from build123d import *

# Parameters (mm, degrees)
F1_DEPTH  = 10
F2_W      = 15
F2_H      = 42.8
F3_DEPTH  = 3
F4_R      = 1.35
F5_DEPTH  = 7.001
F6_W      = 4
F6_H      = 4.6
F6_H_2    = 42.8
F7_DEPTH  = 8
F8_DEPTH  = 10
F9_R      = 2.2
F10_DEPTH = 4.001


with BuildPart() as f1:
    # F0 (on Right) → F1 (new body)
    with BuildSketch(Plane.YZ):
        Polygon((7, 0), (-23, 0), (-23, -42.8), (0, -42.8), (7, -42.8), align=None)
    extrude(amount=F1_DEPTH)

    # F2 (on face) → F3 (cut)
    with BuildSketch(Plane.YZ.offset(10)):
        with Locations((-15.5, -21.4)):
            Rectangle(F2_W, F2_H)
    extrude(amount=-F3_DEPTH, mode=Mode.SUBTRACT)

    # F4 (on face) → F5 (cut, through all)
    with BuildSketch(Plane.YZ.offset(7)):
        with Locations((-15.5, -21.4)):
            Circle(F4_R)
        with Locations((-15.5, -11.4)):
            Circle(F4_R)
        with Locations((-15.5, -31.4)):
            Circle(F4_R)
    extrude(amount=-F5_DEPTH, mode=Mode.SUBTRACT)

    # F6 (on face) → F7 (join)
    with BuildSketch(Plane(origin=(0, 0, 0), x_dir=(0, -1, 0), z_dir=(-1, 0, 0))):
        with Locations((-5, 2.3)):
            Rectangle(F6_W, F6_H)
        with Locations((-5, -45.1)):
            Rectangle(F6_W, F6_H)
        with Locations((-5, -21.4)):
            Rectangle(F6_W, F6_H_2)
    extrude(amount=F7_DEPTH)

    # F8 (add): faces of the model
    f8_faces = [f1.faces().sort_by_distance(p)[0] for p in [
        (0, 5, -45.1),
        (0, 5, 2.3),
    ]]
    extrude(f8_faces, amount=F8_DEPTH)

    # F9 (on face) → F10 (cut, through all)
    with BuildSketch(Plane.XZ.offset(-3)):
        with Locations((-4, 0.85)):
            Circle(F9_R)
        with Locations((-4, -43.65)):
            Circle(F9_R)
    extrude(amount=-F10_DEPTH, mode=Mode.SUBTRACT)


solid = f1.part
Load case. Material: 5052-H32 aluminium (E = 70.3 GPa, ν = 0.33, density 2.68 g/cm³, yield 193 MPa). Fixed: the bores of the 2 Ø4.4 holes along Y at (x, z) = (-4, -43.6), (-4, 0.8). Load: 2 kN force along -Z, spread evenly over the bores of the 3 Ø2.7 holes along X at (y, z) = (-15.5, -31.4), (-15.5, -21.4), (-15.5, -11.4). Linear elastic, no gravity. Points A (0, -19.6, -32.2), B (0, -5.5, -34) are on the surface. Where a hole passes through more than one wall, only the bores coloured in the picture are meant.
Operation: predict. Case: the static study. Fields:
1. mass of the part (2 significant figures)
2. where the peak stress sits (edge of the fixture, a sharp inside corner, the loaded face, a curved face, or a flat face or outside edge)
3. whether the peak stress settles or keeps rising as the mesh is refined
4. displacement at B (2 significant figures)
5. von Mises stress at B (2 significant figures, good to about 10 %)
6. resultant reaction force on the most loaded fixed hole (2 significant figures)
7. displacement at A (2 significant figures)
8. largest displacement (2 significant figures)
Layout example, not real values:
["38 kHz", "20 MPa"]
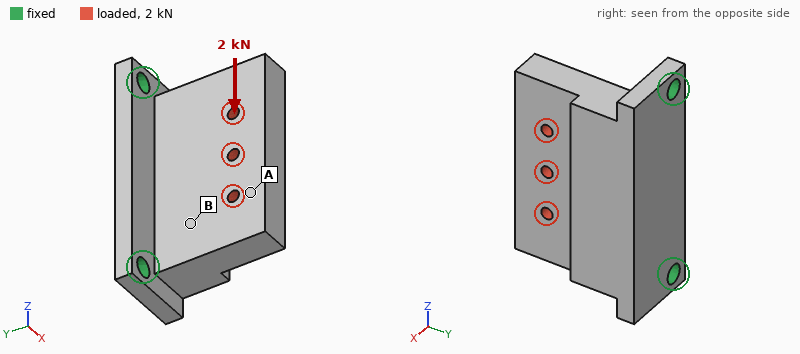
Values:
["34 g", "edge of the fixture", "keeps rising", "16 µm", "24 MPa", "1.4 kN", "29 µm", "36 µm"]
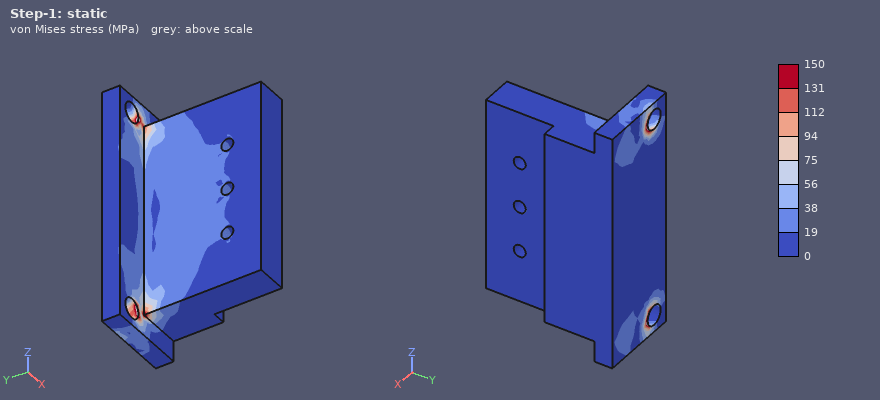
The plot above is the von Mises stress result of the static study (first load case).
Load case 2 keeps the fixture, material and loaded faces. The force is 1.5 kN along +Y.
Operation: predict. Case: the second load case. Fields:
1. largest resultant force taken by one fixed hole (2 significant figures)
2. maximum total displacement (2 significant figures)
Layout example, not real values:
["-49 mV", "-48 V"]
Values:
["770 N", "99 µm"]
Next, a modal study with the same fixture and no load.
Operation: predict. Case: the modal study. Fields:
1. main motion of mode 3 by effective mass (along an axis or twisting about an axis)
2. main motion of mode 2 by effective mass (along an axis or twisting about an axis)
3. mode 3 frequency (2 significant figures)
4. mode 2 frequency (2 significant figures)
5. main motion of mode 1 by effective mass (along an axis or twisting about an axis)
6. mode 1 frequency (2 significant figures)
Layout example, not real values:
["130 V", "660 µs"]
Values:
["along Y", "along Z", "11 kHz", "9600 Hz", "along X", "2600 Hz"]
